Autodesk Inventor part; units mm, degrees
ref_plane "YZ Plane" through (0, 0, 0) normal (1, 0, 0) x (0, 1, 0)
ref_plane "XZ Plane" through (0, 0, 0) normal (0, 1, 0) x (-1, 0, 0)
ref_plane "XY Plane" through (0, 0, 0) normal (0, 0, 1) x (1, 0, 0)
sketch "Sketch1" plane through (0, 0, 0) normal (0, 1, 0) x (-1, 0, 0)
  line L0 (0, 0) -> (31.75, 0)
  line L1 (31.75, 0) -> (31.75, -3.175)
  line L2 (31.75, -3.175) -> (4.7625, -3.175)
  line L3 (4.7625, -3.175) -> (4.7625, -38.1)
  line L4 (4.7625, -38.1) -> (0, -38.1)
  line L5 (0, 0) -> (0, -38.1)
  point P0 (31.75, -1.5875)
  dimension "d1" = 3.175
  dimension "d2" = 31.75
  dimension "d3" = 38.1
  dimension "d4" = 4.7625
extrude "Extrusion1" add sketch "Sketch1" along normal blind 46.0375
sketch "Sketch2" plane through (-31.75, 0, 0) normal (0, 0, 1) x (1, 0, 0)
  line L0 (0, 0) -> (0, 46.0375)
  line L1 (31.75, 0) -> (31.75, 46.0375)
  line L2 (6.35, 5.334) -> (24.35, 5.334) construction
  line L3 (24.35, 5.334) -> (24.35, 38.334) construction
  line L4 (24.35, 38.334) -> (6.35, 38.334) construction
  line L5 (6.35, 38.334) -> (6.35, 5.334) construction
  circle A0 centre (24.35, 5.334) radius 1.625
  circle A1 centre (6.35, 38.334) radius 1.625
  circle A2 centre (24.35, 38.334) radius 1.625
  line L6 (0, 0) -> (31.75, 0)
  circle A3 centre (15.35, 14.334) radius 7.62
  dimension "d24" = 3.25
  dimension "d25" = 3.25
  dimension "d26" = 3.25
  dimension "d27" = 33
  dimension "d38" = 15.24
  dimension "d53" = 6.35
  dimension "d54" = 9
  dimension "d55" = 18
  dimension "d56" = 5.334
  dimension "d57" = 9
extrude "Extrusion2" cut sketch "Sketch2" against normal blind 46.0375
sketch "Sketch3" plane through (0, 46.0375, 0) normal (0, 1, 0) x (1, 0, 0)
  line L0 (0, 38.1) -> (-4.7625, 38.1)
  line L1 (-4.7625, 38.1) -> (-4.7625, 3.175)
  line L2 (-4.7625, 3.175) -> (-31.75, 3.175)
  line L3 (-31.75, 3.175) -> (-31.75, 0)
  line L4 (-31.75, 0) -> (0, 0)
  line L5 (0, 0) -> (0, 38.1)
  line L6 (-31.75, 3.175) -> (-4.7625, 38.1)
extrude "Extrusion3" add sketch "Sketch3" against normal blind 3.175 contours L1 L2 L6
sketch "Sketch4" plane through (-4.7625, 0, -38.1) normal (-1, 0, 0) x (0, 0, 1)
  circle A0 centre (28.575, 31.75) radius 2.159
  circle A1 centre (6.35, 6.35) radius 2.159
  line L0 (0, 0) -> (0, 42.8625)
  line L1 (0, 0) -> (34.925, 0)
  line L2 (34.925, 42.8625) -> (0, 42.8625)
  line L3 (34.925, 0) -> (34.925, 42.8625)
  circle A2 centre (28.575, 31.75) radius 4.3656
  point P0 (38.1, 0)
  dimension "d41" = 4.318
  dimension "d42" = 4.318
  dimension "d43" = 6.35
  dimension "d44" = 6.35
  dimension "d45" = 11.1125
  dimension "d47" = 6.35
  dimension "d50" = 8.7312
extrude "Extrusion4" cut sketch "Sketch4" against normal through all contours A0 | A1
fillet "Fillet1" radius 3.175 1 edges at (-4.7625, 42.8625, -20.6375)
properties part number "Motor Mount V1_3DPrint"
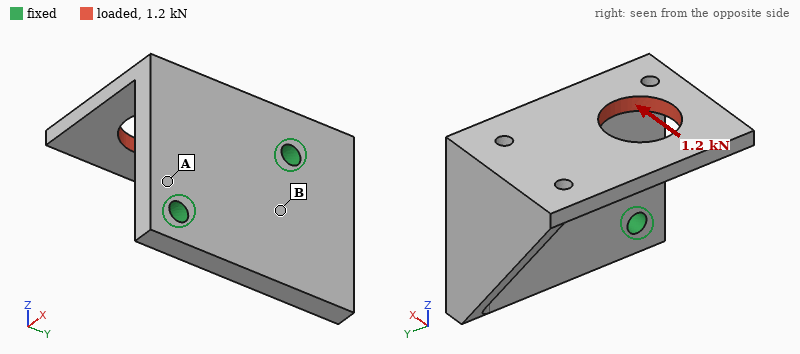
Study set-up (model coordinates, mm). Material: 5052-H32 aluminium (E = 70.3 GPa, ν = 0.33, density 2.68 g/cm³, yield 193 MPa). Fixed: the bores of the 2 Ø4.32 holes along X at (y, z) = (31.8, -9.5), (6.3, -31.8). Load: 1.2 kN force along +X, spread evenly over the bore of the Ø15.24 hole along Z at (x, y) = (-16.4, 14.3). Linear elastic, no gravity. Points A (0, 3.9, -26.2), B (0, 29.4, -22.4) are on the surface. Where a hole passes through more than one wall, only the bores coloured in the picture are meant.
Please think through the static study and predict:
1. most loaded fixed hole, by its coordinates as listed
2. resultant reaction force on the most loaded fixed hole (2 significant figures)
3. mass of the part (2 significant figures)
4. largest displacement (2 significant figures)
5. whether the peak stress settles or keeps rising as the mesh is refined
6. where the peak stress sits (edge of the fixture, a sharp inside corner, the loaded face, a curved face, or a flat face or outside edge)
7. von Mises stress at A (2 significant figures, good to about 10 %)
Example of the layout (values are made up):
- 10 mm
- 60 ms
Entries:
- (31.8, -9.5)
- 980 N
- 35 g
- 0.24 mm
- keeps rising
- edge of the fixture
- 69 MPa
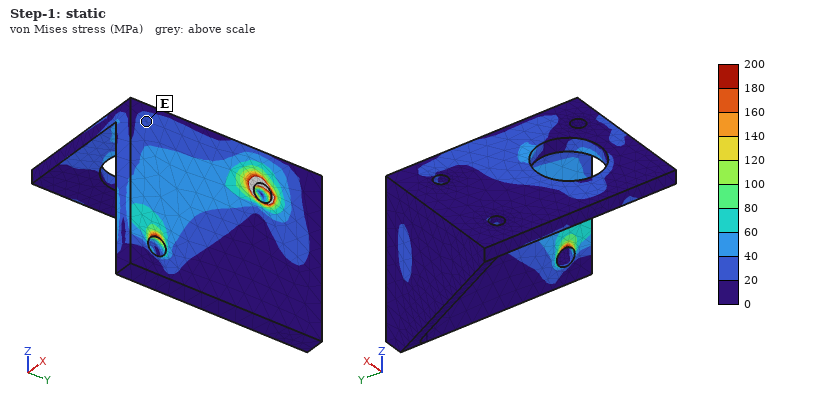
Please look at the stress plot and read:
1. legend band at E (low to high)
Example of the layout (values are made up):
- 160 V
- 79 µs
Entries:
- 20 to 40 MPa
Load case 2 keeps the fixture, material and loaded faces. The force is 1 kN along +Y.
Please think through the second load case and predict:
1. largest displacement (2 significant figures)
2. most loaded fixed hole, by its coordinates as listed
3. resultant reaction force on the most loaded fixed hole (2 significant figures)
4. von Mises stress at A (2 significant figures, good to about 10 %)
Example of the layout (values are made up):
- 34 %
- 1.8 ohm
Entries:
- 0.13 mm
- (31.8, -9.5)
- 1.0 kN
- 44 MPa
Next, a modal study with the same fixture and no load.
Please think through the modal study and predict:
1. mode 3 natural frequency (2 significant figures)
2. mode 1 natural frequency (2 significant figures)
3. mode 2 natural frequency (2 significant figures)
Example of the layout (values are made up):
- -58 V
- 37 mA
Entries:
- 5000 Hz
- 3100 Hz
- 4200 Hz
